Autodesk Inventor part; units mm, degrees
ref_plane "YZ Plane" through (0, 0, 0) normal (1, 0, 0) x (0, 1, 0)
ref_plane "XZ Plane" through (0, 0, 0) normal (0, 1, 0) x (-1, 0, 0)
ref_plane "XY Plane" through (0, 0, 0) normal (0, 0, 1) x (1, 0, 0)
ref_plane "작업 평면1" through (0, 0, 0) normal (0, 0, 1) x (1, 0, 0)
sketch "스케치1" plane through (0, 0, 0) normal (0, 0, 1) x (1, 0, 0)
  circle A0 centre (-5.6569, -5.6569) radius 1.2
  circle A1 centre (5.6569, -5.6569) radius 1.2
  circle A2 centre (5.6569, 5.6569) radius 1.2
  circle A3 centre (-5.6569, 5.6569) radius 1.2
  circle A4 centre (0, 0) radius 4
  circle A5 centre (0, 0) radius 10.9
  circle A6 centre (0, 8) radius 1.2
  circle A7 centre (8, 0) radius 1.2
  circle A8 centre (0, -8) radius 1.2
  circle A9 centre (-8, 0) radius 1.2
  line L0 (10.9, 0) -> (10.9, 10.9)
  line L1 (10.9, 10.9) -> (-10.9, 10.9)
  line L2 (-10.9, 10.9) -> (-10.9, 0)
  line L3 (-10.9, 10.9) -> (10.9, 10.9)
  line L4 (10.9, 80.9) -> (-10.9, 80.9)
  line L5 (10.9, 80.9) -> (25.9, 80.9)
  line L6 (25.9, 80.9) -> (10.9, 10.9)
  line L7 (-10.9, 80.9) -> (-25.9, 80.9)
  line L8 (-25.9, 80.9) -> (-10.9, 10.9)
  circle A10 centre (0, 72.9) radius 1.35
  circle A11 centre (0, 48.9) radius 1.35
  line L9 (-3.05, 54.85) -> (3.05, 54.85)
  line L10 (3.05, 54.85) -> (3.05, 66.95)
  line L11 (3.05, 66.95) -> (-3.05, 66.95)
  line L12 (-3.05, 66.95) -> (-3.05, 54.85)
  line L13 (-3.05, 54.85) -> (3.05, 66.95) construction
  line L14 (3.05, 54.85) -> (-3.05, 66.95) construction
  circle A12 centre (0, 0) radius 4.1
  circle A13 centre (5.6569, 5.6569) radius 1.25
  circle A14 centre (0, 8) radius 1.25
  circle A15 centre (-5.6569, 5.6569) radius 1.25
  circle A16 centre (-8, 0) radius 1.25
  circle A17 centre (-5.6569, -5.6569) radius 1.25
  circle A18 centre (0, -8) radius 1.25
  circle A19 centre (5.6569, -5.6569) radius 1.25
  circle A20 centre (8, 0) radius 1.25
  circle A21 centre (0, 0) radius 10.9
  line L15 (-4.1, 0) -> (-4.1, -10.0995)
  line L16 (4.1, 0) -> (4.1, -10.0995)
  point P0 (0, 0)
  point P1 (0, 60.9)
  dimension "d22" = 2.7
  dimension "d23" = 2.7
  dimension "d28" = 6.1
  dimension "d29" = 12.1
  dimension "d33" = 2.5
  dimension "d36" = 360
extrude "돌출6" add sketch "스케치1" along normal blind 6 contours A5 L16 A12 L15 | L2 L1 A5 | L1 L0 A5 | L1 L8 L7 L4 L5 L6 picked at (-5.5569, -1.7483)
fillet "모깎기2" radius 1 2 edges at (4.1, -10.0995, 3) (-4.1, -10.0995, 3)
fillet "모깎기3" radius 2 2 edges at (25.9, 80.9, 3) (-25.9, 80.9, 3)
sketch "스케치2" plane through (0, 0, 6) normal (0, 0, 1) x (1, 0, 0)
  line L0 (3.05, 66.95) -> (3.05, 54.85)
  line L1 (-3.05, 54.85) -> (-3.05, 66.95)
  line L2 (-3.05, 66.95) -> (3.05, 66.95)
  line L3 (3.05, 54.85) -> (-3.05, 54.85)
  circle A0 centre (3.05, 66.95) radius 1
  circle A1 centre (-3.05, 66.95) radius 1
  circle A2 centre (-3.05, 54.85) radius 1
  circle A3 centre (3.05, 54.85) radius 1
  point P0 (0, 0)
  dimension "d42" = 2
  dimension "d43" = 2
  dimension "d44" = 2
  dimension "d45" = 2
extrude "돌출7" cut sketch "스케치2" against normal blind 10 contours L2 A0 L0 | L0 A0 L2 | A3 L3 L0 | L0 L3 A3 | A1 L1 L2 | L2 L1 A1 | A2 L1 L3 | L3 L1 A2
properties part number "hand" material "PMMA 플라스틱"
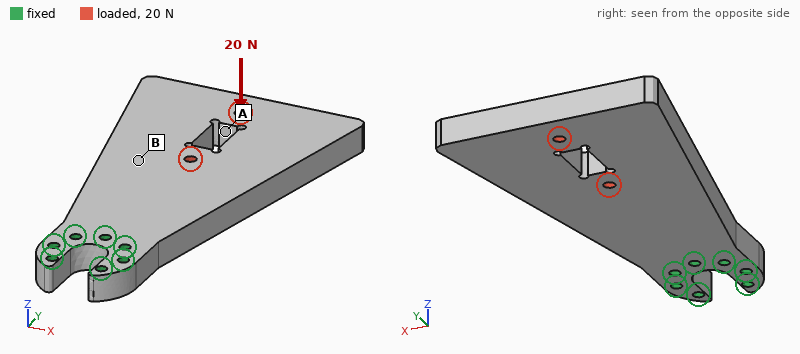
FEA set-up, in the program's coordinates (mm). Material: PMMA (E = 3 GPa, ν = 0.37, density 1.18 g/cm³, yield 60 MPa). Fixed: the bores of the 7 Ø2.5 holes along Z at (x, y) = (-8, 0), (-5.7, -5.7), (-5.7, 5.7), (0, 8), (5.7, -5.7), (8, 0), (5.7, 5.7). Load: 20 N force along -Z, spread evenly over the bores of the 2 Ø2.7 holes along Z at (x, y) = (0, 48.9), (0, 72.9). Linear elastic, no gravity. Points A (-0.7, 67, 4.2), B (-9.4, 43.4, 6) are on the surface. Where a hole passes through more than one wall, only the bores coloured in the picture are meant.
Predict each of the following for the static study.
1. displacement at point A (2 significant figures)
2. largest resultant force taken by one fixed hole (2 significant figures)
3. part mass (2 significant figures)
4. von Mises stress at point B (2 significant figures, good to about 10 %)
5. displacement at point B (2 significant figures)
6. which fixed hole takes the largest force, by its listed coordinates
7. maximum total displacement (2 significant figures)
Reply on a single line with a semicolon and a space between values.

0.86 mm; 55 N; 19 g; 1.7 MPa; 0.41 mm; (0, 8); 1.1 mm
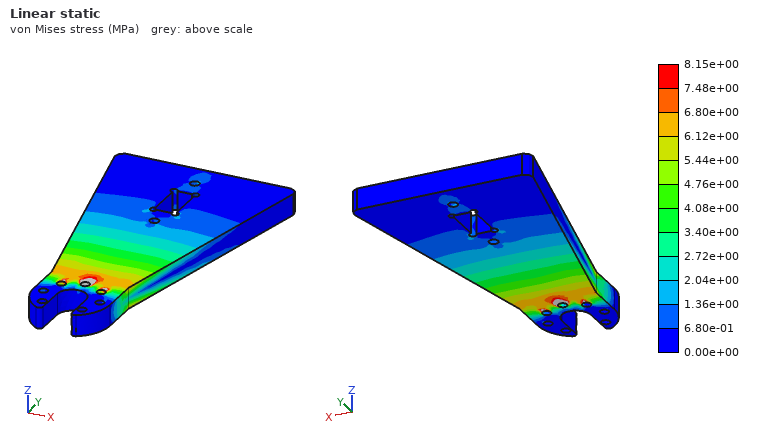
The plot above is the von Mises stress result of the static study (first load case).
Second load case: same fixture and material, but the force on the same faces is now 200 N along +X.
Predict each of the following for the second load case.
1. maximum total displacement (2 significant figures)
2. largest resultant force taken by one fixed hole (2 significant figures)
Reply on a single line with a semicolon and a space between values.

1.0 mm; 510 N
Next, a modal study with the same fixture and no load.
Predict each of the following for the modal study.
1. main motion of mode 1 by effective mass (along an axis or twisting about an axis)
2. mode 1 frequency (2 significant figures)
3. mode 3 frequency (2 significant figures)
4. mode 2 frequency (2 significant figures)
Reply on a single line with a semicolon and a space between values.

along Z; 220 Hz; 720 Hz; 710 Hz
